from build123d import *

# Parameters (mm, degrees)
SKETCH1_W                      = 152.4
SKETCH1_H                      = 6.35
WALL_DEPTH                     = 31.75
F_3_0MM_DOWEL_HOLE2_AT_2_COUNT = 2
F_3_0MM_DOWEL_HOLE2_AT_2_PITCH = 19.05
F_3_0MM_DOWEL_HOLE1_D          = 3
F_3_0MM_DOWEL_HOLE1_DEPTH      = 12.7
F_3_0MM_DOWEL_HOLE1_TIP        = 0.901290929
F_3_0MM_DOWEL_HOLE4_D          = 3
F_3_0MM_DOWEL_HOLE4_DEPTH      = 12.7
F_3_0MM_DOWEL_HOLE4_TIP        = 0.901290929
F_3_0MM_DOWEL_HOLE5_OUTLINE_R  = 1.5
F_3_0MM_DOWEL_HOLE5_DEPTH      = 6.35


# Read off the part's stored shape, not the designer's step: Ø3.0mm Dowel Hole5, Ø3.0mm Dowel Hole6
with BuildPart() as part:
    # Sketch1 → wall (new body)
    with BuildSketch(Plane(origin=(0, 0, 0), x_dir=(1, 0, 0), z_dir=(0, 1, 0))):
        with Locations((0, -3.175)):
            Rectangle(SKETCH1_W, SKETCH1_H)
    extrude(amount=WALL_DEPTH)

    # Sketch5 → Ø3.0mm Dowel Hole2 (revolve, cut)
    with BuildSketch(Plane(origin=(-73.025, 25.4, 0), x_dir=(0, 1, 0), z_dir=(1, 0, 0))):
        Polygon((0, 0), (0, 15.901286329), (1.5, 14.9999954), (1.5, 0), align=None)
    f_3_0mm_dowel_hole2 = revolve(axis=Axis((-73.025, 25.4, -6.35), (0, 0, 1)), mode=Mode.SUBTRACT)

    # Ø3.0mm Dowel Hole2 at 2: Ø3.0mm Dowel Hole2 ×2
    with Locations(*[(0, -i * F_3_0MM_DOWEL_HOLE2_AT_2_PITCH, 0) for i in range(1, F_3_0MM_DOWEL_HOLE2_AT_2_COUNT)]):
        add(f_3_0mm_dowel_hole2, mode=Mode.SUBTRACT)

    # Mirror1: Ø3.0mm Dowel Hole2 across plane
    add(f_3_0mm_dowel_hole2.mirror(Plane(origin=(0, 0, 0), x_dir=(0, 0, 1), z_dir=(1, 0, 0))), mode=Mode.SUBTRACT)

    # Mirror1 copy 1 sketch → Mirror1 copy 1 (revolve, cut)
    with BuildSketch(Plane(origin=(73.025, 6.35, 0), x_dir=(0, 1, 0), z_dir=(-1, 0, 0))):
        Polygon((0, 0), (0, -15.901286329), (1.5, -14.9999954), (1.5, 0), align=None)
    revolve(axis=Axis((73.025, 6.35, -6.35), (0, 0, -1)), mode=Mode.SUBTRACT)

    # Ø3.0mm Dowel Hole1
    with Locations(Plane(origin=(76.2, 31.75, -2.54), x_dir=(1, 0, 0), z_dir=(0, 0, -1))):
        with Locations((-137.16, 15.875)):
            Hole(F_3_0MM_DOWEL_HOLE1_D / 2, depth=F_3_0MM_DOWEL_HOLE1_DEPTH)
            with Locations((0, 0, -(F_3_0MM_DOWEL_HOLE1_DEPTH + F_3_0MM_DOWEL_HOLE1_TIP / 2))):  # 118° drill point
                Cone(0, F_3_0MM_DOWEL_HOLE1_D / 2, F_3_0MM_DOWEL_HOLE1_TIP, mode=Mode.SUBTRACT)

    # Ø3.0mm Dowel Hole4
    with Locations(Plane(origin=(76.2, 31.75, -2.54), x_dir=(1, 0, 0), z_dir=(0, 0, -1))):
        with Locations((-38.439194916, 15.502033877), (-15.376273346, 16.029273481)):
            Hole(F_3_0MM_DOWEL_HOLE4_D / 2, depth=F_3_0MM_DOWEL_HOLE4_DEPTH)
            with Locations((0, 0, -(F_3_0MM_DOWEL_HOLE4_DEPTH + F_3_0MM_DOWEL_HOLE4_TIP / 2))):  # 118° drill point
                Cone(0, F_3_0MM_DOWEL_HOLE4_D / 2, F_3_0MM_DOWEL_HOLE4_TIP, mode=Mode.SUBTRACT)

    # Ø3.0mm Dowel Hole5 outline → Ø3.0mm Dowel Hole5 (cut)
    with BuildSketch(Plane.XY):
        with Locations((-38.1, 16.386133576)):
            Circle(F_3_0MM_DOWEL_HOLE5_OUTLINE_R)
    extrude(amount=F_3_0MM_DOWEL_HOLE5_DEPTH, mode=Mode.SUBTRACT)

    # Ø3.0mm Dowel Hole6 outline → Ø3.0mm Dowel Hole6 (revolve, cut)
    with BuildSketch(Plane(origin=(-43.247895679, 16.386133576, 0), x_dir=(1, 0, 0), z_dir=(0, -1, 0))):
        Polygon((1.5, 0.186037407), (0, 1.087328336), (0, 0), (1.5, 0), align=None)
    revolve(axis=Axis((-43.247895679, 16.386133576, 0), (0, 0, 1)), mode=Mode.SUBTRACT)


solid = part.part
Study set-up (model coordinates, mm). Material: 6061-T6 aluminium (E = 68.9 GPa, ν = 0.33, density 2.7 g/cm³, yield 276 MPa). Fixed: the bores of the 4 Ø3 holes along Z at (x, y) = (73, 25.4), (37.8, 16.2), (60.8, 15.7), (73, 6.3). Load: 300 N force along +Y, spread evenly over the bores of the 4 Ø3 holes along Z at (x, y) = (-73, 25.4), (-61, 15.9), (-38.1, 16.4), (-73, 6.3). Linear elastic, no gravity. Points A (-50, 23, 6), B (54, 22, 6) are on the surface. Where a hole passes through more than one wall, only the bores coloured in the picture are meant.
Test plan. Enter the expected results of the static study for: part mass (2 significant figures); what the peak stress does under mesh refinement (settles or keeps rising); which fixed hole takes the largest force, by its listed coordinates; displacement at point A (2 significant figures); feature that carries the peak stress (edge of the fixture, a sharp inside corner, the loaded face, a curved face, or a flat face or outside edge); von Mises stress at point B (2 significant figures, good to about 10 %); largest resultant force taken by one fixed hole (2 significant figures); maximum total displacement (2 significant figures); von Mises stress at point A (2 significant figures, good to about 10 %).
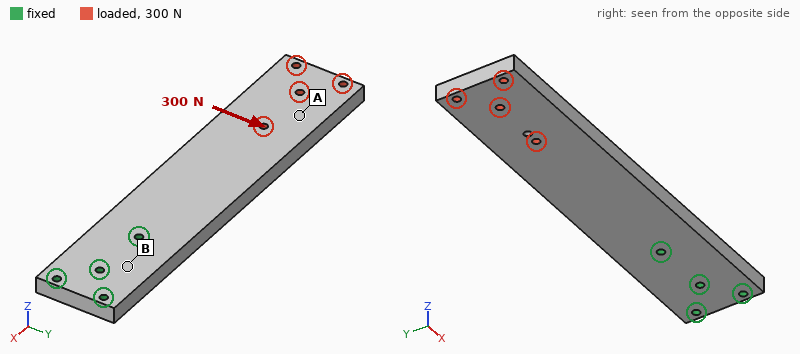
82 g
keeps rising
(37.8, 16.2)
0.11 mm
edge of the fixture
11 MPa
1.1 kN
0.16 mm
3.0 MPa
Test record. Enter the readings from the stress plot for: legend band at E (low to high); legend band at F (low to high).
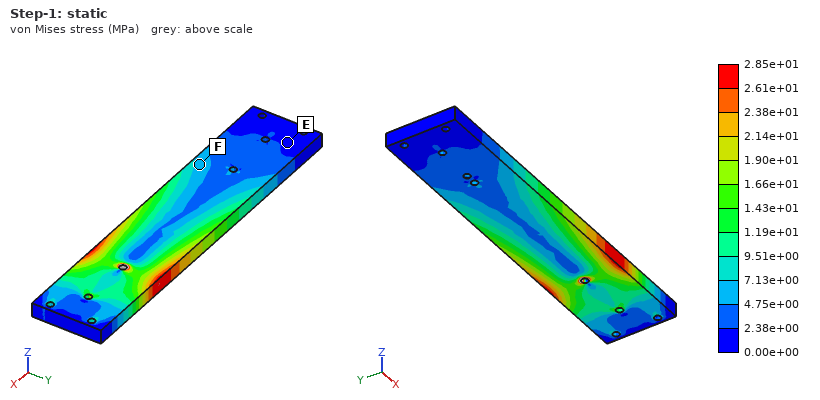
0.00e+00 to 2.38e+00 MPa
4.75e+00 to 7.13e+00 MPa
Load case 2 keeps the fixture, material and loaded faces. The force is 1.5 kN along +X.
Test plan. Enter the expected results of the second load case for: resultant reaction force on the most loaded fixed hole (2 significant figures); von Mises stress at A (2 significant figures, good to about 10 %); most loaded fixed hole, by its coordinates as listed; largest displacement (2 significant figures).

1.0 kN
5.8 MPa
(37.8, 16.2)
13 µm
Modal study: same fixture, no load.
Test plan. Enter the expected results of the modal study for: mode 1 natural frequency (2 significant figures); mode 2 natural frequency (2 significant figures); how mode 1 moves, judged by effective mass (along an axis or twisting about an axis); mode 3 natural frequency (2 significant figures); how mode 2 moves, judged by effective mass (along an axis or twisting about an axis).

390 Hz
1500 Hz
along Z
2400 Hz
along Y
